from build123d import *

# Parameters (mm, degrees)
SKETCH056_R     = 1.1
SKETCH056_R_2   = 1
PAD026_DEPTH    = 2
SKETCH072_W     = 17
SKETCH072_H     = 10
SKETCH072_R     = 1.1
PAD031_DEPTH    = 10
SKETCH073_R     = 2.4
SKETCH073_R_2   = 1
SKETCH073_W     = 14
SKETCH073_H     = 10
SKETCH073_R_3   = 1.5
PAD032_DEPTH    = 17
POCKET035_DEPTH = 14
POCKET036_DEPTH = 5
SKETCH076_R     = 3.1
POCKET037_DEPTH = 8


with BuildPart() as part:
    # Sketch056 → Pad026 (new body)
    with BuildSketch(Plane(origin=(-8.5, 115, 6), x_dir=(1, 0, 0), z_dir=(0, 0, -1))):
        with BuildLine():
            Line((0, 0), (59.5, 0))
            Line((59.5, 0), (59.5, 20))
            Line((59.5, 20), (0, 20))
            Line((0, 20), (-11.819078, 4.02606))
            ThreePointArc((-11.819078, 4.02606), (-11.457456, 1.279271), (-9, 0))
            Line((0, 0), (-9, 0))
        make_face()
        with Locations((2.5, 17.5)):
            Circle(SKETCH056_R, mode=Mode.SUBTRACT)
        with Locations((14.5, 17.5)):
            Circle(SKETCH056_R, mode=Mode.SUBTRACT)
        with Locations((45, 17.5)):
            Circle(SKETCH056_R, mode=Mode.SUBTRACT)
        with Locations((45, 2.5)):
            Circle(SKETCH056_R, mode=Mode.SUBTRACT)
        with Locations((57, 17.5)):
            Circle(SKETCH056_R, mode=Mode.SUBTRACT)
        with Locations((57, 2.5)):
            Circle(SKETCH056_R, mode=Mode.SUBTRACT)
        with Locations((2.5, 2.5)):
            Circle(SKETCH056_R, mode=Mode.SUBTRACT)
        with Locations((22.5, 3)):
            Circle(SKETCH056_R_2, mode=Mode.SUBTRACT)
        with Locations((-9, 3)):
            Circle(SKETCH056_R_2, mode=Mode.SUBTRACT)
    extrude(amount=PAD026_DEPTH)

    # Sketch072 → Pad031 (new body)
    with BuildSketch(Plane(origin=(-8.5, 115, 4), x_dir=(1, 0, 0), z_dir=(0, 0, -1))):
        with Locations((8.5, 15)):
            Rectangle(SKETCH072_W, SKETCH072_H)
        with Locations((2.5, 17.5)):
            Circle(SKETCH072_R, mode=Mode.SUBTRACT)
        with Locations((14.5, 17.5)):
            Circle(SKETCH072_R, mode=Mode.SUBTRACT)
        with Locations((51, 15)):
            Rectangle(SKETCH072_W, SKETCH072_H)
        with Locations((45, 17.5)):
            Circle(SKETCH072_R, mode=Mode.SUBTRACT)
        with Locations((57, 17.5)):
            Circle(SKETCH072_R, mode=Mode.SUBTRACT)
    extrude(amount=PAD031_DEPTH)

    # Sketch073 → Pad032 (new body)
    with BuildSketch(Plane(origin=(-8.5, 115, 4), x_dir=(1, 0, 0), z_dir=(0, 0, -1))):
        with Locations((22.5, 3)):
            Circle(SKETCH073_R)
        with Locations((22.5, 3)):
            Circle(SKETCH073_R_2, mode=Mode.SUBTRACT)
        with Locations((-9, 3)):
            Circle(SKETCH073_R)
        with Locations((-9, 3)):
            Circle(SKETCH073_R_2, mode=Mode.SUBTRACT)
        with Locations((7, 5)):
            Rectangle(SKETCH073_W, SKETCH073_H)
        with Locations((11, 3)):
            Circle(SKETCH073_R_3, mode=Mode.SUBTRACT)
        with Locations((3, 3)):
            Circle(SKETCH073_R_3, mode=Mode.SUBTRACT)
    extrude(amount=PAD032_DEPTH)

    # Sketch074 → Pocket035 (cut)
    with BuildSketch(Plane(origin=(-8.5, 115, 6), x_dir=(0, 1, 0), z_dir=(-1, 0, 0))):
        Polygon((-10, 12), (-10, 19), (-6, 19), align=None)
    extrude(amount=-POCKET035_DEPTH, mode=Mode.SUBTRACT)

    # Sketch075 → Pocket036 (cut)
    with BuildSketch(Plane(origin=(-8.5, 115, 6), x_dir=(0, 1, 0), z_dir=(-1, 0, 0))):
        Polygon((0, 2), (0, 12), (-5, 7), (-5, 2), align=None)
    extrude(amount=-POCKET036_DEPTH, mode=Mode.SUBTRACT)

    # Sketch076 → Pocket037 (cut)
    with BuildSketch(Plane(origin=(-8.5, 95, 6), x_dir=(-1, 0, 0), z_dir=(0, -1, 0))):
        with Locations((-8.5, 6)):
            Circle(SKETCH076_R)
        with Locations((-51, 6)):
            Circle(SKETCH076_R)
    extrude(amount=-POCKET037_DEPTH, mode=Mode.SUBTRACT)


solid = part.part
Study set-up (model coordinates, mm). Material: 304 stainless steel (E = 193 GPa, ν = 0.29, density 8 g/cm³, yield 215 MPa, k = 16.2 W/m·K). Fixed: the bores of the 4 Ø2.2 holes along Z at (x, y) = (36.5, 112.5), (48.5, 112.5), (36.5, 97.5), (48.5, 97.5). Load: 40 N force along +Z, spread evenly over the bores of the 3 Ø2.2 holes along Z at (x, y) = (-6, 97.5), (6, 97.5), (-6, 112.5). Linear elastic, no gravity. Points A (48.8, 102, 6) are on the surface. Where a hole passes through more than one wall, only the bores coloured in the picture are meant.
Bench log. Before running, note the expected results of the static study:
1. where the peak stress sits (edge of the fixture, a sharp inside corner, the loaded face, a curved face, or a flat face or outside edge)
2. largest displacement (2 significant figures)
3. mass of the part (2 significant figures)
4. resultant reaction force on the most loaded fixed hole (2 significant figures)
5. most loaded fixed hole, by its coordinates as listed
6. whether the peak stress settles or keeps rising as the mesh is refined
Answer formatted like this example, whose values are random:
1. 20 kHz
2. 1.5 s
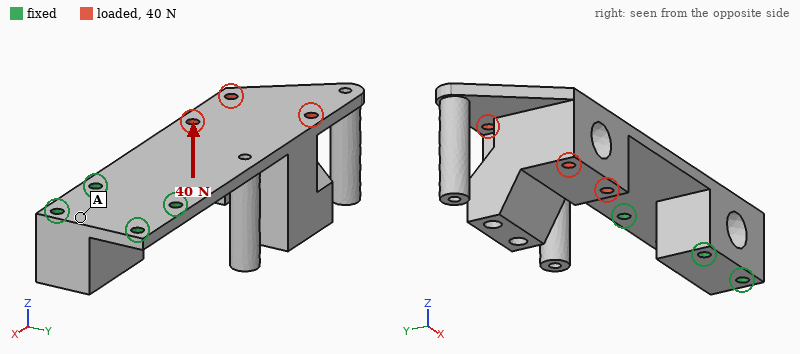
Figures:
1. edge of the fixture
2. 0.43 mm
3. 61 g
4. 75 N
5. (36.5, 97.5)
6. keeps rising
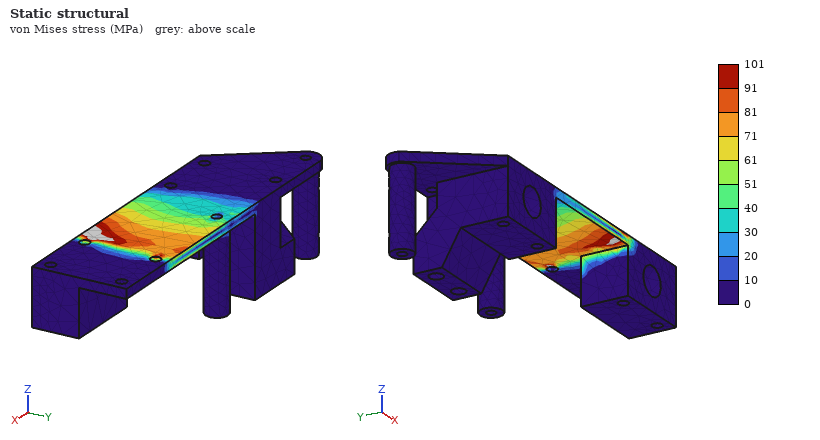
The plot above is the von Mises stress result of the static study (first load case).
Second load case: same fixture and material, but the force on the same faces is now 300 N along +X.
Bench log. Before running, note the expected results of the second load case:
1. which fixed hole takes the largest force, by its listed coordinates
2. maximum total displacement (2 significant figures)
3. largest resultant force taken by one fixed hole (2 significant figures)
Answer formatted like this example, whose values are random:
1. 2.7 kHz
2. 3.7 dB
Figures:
1. (36.5, 97.5)
2. 0.65 mm
3. 260 N
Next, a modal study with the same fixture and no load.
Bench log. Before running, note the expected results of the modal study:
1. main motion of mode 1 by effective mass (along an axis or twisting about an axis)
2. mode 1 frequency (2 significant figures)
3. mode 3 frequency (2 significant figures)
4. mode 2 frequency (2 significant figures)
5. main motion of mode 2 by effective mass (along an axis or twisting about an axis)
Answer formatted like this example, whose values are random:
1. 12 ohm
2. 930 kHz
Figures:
1. along Z
2. 300 Hz
3. 2100 Hz
4. 1100 Hz
5. along Y
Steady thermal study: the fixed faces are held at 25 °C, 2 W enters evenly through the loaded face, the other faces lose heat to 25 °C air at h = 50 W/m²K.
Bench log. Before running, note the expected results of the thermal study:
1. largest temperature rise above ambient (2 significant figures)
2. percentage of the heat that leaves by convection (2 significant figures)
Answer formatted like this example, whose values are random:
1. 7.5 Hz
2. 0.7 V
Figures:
1. 16 K
2. 93 %
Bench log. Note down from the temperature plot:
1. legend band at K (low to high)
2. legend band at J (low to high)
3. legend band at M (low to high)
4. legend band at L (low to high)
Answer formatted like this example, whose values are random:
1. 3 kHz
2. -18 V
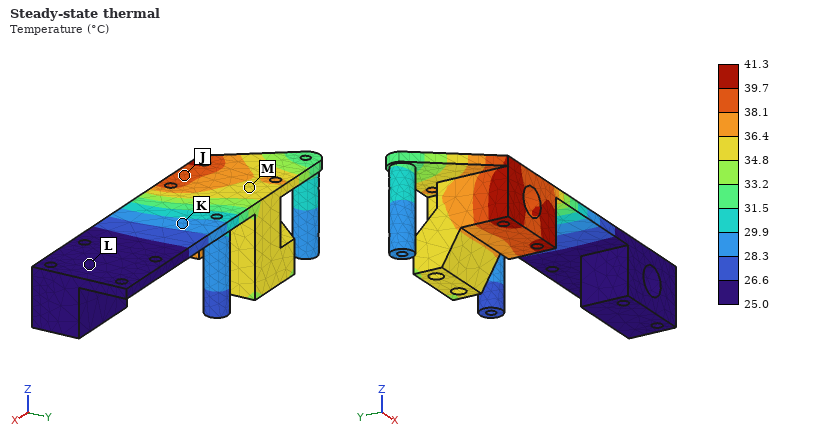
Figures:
1. 28.3 to 29.9 °C
2. 38.1 to 39.7 °C
3. 34.8 to 36.4 °C
4. 25.0 to 26.6 °C
